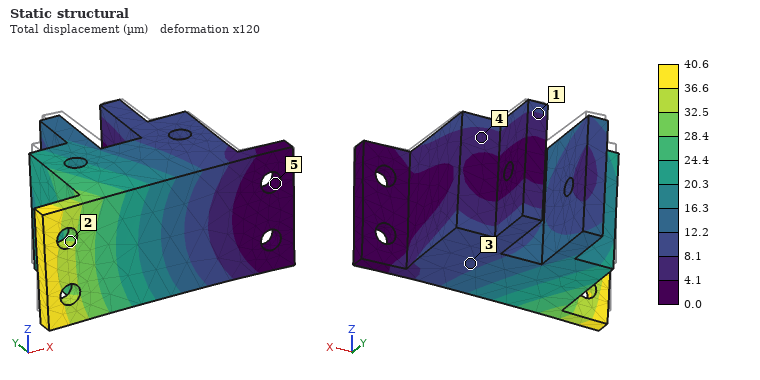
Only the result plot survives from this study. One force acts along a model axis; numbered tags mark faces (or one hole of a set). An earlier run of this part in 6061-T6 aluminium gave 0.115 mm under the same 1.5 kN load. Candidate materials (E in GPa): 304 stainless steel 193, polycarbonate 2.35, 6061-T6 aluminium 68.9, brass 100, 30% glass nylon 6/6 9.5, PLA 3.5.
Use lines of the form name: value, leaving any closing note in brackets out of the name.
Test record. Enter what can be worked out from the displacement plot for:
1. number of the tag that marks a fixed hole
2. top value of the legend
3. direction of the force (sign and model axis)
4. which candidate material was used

number of the tag that marks a fixed hole: 5
top value of the legend: 40.6 µm
direction of the force: -Z
which candidate material was used: 304 stainless steel
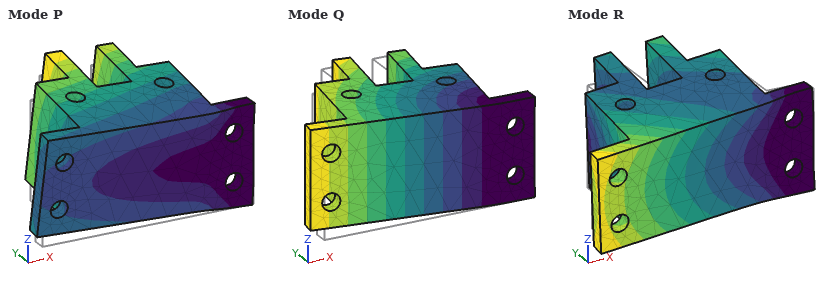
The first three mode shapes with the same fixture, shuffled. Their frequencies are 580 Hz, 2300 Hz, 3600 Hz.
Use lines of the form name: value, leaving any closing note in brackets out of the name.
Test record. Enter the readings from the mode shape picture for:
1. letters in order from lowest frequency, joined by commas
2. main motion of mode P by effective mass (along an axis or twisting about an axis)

letters in order from lowest frequency, joined by commas: Q, P, R
main motion of mode P by effective mass: along Z
